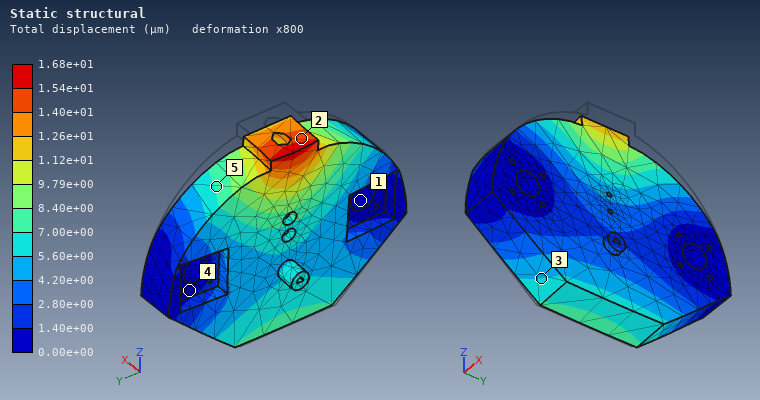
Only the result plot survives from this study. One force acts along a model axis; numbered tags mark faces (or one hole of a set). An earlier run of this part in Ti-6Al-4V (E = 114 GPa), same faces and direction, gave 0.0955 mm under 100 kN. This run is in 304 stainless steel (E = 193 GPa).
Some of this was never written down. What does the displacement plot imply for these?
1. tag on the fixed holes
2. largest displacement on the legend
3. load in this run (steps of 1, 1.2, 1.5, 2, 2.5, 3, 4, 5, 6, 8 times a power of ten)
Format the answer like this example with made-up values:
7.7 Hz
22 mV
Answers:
1
1.68e+01 µm
30 kN
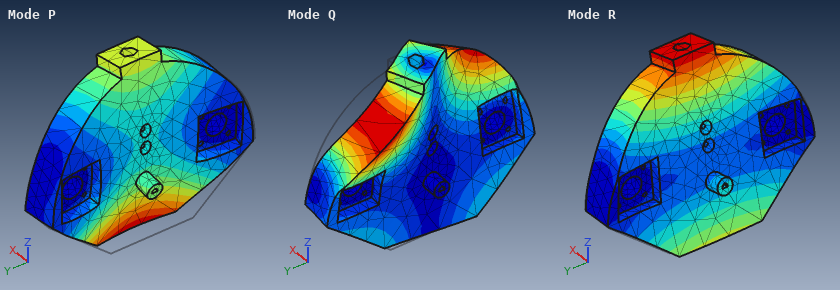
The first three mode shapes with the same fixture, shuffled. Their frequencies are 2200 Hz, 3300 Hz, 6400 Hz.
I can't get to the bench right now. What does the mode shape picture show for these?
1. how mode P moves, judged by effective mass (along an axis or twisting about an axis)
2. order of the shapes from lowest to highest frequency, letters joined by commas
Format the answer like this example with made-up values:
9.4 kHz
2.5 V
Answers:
along X
R, P, Q
